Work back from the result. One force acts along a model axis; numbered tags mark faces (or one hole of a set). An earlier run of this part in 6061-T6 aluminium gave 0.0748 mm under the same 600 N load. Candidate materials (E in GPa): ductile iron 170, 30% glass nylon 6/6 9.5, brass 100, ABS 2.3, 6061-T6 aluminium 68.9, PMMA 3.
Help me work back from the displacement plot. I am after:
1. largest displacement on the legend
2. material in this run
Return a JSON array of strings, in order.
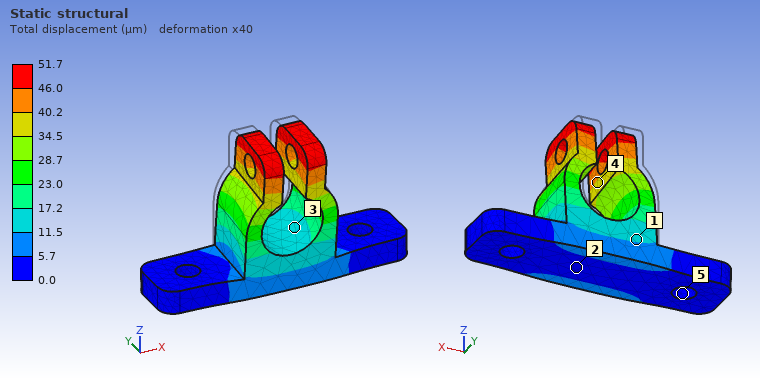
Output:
["51.7 µm", "brass"]
